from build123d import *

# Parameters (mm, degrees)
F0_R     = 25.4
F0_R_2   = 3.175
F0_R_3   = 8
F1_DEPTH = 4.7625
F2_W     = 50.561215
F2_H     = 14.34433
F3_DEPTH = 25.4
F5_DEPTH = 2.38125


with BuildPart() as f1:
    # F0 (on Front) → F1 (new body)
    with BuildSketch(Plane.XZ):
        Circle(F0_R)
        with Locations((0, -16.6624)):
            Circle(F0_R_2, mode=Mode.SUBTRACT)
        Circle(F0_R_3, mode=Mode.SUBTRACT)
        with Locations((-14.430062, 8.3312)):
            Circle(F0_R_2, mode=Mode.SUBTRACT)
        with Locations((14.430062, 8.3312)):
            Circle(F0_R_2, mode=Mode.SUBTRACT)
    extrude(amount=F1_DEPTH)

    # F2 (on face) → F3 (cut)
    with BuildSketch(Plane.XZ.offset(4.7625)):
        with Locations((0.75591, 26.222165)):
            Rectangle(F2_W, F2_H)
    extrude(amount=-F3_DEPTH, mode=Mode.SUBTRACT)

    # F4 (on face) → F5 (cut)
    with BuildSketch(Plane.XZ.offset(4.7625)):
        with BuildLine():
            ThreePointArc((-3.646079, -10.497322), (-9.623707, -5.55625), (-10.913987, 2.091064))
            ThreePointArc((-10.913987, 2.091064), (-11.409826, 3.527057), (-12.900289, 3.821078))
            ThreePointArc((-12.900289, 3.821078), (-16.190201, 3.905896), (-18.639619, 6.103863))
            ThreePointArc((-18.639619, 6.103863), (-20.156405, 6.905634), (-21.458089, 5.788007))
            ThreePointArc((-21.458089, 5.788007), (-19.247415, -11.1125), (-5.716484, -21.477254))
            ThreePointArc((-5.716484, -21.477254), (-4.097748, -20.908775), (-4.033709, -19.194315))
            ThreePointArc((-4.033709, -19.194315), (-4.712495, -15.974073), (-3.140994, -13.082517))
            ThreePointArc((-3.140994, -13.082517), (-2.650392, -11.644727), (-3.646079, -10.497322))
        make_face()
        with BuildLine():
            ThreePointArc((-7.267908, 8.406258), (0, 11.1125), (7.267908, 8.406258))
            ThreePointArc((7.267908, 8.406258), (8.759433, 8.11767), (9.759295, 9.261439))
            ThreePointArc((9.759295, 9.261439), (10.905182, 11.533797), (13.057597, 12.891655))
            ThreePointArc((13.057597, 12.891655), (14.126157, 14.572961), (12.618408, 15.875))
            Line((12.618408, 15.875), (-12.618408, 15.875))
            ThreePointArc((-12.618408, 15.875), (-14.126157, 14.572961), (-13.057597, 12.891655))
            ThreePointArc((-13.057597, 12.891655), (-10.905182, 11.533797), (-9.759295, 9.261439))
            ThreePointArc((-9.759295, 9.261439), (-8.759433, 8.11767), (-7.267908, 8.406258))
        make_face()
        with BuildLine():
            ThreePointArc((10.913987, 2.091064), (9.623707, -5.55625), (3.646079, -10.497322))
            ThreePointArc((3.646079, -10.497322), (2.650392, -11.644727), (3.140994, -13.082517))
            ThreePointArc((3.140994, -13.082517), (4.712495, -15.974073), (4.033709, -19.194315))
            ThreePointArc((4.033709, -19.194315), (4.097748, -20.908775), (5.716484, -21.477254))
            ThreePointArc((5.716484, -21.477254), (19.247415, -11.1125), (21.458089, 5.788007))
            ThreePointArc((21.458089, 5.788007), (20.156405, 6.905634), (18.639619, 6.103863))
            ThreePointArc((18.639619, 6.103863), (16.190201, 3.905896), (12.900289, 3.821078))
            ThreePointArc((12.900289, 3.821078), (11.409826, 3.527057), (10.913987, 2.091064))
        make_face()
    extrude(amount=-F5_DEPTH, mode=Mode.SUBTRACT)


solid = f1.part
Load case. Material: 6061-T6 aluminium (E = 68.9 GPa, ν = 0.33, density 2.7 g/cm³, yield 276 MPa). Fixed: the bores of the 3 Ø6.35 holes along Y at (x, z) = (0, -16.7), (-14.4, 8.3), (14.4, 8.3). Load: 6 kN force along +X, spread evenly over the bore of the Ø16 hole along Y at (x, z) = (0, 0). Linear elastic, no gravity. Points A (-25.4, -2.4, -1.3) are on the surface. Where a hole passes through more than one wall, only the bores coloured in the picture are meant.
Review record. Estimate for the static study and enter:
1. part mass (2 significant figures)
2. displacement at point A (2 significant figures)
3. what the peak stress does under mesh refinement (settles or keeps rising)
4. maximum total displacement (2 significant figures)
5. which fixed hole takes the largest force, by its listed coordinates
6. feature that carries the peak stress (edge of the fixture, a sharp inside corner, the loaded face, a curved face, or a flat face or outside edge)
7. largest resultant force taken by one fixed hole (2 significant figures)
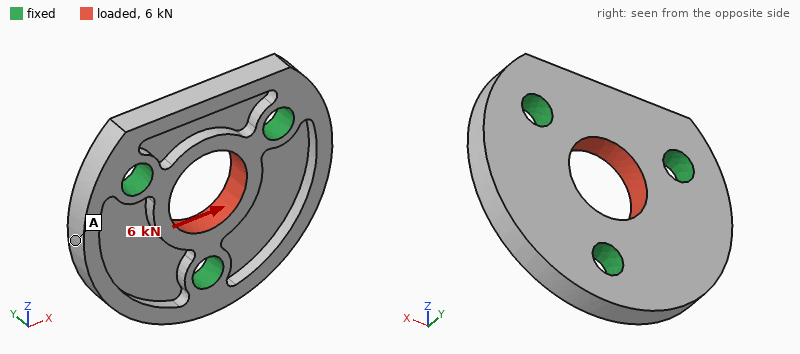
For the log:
16 g
3.9 µm
keeps rising
17 µm
(0, -16.7)
edge of the fixture
2.2 kN
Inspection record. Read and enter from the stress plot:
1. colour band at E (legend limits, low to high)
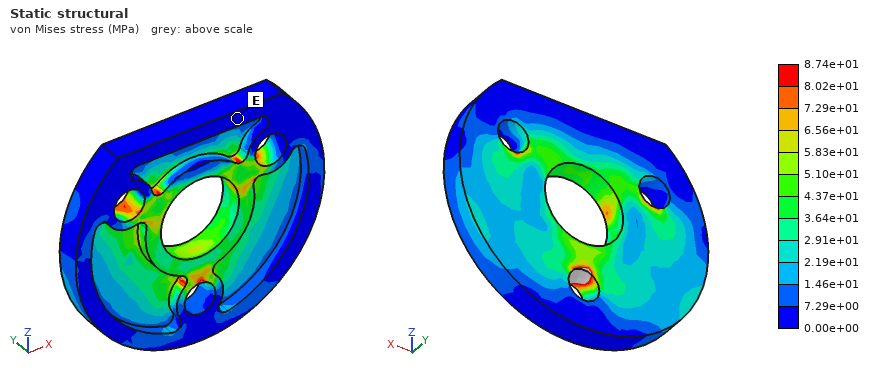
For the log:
0.00e+00 to 7.29e+00 MPa
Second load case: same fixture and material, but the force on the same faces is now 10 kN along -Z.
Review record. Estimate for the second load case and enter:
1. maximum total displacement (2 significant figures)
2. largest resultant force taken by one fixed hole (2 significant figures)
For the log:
34 µm
3.5 kN
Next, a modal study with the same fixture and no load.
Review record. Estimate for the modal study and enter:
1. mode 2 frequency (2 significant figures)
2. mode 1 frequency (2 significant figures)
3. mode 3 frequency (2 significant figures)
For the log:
11 kHz
11 kHz
21 kHz
